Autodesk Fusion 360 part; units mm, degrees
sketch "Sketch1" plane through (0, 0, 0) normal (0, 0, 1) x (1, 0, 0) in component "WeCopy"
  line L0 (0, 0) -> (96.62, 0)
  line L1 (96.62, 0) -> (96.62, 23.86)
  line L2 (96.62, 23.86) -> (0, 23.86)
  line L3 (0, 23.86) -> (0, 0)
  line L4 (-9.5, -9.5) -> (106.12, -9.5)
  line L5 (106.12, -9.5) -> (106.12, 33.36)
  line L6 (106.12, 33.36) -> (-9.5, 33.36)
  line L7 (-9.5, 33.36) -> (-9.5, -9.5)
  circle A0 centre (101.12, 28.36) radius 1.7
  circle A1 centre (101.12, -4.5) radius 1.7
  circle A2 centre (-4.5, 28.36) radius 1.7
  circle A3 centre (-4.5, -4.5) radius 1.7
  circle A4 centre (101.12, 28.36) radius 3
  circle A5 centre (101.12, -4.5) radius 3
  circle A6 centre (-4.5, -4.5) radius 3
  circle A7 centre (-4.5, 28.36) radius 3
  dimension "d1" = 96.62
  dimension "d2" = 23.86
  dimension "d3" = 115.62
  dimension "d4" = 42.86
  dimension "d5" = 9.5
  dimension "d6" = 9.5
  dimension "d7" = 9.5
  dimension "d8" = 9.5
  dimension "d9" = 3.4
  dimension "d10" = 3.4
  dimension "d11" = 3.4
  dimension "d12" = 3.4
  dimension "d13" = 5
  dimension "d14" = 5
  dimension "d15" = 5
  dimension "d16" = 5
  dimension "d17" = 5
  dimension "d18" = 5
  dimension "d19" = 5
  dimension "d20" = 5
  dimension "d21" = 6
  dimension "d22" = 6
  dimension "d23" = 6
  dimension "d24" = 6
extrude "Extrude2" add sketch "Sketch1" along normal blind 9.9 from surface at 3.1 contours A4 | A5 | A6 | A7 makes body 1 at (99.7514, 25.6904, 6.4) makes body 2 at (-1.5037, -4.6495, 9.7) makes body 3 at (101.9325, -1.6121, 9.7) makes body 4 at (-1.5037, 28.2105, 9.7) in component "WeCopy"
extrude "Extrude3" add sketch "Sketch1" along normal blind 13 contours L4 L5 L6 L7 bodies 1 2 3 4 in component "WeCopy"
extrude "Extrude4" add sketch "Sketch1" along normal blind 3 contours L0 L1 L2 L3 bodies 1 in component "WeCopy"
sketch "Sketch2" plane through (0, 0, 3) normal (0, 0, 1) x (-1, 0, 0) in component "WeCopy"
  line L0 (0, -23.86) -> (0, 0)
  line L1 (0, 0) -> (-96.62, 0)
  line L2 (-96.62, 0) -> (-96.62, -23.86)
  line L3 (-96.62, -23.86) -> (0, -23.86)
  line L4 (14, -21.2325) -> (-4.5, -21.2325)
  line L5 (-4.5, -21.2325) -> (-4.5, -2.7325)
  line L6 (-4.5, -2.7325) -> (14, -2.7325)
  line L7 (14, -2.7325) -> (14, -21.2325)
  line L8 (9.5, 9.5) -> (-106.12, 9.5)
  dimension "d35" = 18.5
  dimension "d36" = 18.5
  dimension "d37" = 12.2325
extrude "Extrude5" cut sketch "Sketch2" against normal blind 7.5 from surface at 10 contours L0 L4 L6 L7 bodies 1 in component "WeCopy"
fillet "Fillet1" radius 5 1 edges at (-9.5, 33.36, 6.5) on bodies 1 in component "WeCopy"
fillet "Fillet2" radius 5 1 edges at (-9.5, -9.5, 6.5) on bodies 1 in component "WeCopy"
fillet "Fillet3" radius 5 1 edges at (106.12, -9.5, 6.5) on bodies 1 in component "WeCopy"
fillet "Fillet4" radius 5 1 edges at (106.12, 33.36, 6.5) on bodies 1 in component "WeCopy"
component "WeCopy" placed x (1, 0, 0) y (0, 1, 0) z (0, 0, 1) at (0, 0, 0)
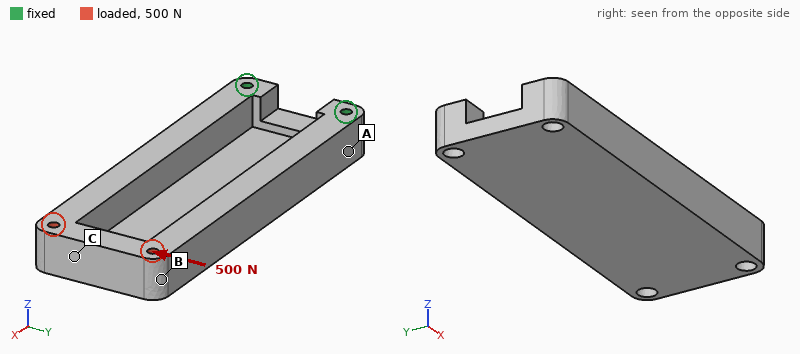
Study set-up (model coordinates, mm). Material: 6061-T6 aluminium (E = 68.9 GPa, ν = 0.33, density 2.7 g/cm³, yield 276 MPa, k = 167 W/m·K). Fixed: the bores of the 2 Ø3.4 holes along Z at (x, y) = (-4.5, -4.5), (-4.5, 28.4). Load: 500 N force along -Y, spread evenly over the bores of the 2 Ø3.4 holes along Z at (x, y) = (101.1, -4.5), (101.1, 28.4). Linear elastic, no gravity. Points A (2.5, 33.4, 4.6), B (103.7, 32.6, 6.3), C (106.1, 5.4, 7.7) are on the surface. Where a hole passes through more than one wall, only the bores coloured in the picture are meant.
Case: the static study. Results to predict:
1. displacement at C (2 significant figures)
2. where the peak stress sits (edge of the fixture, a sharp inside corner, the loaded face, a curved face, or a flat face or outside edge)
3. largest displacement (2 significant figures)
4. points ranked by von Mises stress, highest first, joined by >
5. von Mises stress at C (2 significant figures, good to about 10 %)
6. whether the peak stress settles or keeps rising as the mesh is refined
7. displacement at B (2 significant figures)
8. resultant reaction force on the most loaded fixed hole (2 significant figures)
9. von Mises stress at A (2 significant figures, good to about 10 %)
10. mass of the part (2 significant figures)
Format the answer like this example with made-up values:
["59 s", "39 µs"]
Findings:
["0.093 mm", "edge of the fixture", "0.12 mm", "A > C > B", "8.8 MPa", "keeps rising", "0.11 mm", "1.5 kN", "22 MPa", "110 g"]
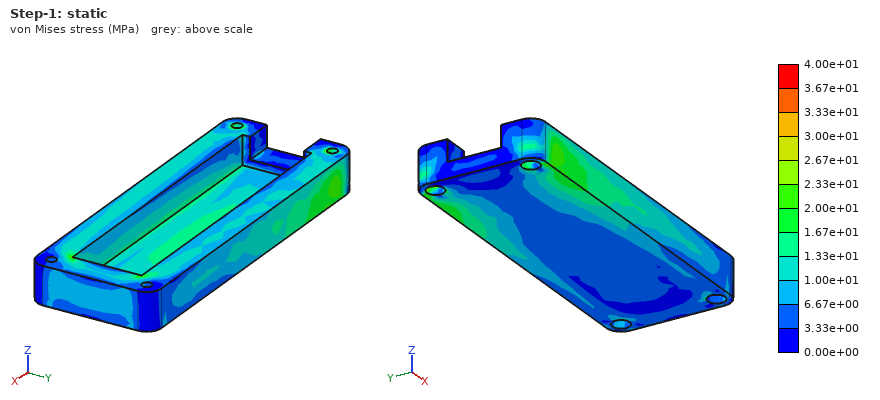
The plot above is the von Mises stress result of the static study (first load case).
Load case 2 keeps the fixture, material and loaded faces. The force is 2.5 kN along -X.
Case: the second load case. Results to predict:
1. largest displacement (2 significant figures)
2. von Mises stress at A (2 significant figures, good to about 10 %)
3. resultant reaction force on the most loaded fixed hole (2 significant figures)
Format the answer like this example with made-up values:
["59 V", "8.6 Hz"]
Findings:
["0.11 mm", "7.3 MPa", "1.3 kN"]
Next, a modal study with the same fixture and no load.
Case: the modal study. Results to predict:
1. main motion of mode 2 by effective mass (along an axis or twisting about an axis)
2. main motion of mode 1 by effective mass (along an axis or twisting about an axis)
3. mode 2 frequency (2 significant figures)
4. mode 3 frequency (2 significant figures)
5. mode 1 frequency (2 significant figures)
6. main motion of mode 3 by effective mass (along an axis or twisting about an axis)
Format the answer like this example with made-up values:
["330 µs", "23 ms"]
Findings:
["along Y", "along Z", "1700 Hz", "3000 Hz", "740 Hz", "along Y"]
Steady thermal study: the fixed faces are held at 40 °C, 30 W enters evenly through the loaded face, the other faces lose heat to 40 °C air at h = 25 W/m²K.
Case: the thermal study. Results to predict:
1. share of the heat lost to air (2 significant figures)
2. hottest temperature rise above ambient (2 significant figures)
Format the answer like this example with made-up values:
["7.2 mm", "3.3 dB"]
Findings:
["31 %", "49 K"]
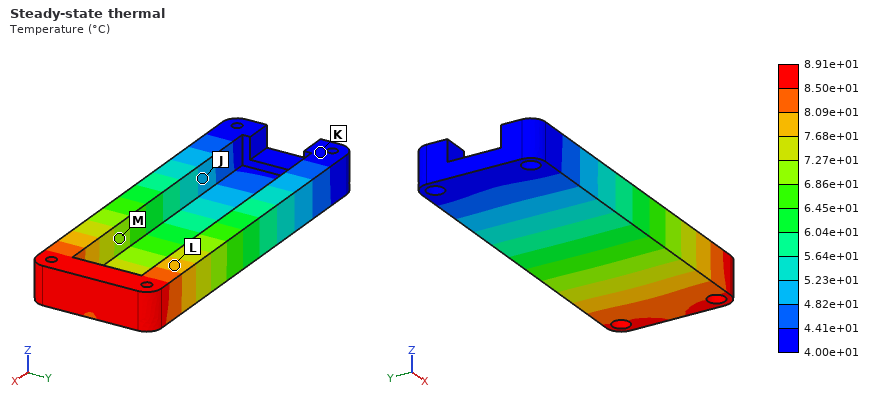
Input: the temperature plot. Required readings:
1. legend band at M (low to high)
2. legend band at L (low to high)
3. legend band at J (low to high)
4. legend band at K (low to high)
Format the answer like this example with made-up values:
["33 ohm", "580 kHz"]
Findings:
["6.86e+01 to 7.27e+01 °C", "7.68e+01 to 8.09e+01 °C", "4.82e+01 to 5.23e+01 °C", "4.00e+01 to 4.41e+01 °C"]
